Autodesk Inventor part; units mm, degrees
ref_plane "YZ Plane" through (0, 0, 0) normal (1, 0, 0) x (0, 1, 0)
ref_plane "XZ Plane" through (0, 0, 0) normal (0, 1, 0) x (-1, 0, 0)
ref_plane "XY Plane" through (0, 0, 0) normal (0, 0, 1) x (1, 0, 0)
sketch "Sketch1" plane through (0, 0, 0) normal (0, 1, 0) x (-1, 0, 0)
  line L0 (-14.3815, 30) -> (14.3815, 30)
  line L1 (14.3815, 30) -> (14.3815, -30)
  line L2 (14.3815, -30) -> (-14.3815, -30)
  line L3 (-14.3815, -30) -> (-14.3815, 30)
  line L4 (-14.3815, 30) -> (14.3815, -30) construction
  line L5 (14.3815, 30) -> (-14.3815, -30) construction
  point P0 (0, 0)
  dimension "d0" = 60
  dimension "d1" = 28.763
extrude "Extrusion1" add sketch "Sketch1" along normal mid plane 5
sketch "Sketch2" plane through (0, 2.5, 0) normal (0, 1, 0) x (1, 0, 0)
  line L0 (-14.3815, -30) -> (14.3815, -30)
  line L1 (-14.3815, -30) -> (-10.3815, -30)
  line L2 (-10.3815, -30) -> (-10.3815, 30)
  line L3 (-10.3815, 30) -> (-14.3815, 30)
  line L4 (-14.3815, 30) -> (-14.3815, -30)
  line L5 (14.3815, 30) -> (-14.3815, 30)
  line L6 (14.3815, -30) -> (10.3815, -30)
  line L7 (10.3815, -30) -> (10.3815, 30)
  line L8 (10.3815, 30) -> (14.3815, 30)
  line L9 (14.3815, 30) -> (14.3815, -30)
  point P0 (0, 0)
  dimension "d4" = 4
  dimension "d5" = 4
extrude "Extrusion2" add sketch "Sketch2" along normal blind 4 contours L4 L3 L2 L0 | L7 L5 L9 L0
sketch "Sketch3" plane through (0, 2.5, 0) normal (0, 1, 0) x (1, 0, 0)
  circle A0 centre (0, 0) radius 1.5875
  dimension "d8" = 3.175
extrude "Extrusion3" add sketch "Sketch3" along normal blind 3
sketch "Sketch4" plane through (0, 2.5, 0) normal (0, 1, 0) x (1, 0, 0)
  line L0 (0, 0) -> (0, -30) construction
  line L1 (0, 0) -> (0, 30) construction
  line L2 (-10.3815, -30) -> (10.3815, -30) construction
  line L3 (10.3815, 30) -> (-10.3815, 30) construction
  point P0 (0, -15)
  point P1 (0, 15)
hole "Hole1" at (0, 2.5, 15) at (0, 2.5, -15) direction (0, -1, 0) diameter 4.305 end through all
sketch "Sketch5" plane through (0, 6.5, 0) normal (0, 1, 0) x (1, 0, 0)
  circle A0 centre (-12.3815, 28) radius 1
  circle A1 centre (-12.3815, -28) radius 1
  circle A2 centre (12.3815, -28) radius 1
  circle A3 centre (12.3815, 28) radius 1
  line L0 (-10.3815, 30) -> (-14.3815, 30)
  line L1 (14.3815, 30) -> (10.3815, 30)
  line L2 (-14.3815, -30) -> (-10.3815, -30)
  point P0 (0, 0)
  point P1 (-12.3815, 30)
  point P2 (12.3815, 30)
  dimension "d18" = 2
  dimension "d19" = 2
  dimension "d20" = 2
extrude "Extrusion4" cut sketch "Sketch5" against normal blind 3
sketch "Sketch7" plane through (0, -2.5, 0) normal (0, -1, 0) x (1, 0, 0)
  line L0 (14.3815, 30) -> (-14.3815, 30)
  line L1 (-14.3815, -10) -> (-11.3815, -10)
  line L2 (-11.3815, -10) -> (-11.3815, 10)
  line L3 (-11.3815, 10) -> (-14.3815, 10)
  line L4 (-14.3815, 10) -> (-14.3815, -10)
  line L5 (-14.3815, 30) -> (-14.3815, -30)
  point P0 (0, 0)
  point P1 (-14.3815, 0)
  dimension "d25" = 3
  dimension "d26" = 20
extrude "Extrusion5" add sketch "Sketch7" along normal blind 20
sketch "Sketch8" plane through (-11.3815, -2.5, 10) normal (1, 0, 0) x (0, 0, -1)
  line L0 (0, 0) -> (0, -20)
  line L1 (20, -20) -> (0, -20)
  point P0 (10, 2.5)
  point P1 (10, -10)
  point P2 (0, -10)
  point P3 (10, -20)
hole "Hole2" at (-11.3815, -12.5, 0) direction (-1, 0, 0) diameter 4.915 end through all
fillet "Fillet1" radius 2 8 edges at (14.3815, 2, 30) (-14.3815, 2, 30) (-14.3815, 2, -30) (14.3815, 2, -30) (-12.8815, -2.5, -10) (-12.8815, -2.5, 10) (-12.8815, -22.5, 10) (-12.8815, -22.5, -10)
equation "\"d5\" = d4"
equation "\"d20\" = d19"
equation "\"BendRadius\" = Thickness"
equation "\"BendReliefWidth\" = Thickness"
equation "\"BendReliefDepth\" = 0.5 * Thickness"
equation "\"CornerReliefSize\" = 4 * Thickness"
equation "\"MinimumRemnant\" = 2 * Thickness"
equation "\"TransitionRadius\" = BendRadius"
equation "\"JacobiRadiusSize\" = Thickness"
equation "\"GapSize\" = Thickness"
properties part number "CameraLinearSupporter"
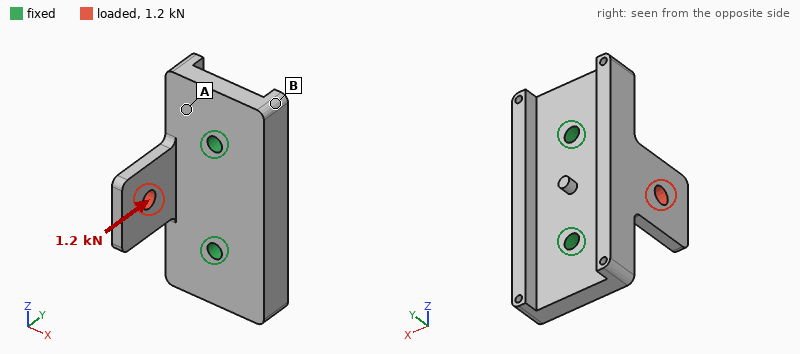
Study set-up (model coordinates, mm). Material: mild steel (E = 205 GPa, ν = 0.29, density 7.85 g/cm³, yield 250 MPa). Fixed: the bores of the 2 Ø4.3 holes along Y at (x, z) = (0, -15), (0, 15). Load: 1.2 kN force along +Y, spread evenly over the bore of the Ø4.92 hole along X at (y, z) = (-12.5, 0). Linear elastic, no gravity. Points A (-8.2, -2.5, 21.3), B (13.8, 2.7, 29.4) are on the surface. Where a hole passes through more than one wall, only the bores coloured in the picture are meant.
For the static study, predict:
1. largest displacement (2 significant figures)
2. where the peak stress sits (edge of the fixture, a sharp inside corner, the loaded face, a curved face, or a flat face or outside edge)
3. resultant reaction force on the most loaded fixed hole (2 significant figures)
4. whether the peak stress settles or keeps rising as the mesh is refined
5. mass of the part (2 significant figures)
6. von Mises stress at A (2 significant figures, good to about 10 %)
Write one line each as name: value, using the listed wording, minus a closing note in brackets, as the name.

largest displacement: 31 µm
where the peak stress sits: edge of the fixture
resultant reaction force on the most loaded fixed hole: 600 N
whether the peak stress settles or keeps rising as the mesh is refined: keeps rising
mass of the part: 90 g
von Mises stress at A: 26 MPa
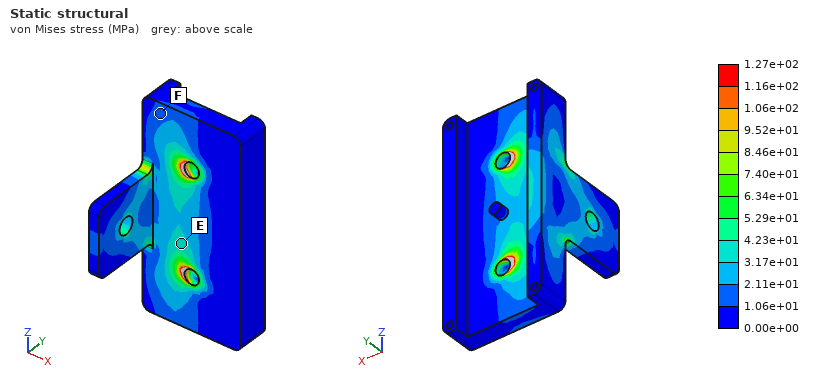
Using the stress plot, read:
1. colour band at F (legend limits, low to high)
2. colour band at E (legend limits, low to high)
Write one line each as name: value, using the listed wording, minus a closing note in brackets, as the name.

colour band at F: 1.06e+01 to 2.11e+01 MPa
colour band at E: 3.17e+01 to 4.23e+01 MPa
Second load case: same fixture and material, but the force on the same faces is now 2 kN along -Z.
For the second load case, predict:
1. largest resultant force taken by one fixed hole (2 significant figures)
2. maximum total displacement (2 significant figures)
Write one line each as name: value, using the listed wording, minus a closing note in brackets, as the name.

largest resultant force taken by one fixed hole: 1.5 kN
maximum total displacement: 35 µm
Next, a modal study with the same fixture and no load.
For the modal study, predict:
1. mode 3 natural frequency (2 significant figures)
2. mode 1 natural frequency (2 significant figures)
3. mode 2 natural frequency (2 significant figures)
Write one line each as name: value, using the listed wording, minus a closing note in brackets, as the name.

mode 3 natural frequency: 11 kHz
mode 1 natural frequency: 4800 Hz
mode 2 natural frequency: 9900 Hz
